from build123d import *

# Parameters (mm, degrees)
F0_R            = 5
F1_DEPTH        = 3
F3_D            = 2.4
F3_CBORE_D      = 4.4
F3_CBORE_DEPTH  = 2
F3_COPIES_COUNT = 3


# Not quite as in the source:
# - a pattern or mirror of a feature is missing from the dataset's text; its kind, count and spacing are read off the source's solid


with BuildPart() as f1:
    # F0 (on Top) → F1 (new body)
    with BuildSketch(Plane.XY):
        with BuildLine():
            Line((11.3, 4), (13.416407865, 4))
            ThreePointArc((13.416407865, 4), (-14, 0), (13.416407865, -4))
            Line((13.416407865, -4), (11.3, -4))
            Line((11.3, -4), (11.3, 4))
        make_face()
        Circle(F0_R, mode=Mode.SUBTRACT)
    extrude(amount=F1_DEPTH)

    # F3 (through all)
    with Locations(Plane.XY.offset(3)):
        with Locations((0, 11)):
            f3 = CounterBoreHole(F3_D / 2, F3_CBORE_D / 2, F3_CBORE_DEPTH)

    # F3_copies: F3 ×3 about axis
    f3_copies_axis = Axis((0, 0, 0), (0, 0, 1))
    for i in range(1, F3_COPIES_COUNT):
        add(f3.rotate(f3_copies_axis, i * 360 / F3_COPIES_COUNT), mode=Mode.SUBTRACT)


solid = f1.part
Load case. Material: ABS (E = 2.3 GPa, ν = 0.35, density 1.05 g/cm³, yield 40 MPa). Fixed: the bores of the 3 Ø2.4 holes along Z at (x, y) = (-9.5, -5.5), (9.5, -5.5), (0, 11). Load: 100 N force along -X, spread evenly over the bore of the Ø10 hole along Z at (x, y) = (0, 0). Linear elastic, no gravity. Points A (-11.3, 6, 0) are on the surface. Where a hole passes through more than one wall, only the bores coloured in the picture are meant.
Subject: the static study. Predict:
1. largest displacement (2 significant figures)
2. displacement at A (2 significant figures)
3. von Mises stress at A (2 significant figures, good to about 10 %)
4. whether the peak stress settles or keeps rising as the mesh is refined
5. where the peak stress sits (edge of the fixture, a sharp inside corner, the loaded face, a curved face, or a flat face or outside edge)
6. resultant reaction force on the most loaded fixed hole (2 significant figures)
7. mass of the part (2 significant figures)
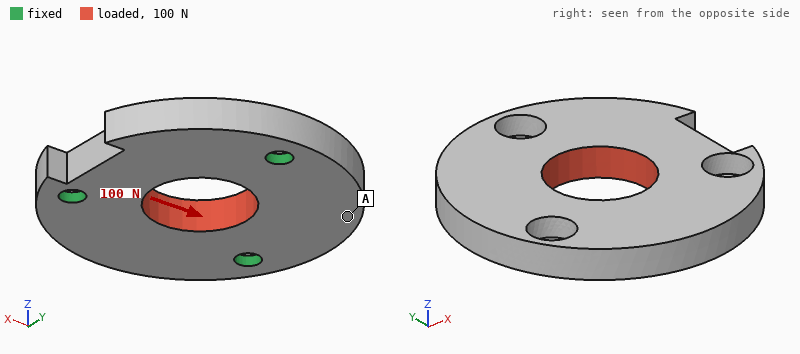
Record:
26 µm
20 µm
1.1 MPa
keeps rising
edge of the fixture
34 N
1.5 g
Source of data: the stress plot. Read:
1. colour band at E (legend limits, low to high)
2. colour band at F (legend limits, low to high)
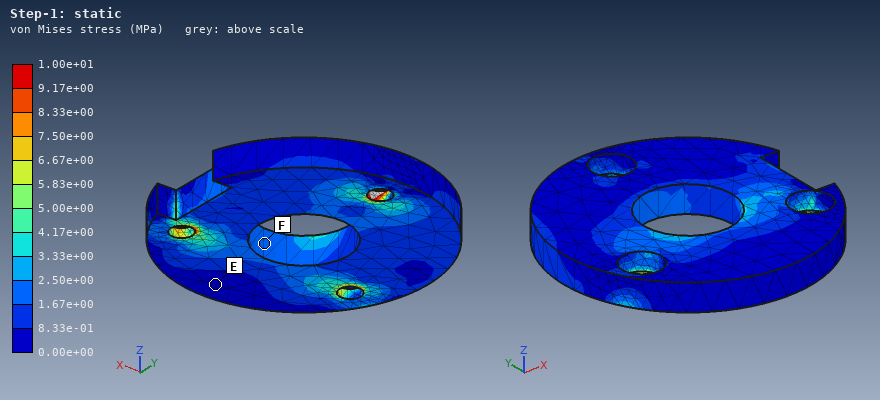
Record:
0.00e+00 to 8.33e-01 MPa
1.67e+00 to 2.50e+00 MPa
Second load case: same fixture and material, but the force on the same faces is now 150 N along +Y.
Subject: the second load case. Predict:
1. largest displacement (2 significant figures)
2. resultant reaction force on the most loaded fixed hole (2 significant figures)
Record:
47 µm
51 N
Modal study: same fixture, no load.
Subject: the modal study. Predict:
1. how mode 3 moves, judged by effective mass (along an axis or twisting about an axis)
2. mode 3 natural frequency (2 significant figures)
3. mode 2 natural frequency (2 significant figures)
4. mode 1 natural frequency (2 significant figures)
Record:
along Z
6500 Hz
4900 Hz
4700 Hz
